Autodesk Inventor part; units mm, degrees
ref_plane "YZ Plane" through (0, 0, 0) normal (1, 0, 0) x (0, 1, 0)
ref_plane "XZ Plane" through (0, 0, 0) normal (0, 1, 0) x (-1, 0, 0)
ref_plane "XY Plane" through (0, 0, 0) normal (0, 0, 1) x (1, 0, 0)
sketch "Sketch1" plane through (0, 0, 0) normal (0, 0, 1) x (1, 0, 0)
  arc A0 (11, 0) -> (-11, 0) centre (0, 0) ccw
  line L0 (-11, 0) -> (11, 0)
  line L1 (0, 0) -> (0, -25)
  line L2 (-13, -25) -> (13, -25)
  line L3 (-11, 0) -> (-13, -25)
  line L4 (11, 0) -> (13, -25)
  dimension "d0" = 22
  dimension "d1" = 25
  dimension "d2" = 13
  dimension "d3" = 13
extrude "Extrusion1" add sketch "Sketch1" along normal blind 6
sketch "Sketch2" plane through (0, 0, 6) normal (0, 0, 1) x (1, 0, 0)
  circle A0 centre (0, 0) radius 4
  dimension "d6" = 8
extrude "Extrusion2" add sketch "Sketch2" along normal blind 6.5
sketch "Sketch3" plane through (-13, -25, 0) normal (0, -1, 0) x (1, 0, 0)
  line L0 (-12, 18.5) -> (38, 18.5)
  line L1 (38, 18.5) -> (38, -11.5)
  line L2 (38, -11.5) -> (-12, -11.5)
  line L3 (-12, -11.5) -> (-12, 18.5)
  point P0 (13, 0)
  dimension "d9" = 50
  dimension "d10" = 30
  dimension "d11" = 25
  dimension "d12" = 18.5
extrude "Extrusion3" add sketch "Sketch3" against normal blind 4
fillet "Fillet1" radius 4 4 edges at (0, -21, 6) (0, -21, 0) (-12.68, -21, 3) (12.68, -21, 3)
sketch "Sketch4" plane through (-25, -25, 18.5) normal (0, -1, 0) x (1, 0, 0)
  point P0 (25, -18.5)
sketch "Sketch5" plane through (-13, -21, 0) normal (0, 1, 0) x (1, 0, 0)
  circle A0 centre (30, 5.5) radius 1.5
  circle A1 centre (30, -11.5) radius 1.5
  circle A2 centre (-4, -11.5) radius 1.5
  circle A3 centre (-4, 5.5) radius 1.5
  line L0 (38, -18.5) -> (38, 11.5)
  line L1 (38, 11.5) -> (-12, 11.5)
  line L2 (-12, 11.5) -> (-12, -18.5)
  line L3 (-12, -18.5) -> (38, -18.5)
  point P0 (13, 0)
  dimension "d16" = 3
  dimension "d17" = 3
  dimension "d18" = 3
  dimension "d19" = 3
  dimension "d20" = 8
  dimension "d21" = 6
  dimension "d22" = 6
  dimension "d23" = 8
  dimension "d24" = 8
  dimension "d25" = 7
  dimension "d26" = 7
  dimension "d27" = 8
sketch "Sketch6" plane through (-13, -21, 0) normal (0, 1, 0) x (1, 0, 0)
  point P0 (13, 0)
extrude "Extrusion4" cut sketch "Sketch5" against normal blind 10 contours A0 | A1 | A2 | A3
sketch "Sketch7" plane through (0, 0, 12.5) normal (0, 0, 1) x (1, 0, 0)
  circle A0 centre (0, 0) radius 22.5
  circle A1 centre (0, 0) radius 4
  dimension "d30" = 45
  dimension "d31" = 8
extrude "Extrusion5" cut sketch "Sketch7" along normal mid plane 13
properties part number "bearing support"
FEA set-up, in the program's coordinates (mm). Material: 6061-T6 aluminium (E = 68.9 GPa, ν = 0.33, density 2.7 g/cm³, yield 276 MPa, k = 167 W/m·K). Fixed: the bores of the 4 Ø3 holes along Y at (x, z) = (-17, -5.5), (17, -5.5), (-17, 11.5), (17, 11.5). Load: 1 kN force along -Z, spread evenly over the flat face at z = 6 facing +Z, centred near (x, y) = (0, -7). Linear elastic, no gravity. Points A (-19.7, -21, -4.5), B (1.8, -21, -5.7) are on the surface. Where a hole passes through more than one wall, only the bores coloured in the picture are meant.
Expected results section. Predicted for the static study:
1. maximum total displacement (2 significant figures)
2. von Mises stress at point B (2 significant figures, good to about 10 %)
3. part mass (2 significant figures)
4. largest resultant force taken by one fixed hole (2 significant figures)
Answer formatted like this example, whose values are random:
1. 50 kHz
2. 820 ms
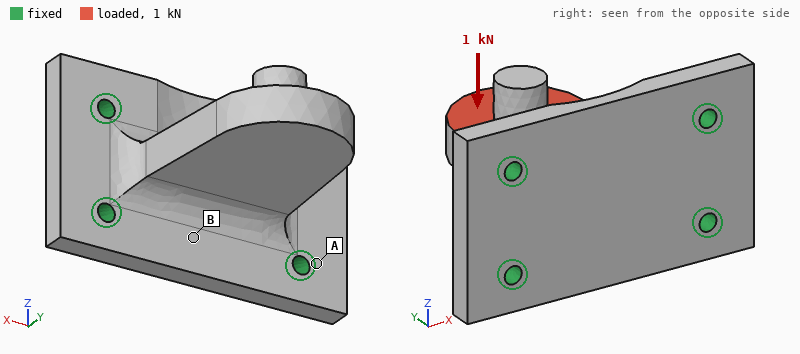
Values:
1. 0.17 mm
2. 22 MPa
3. 28 g
4. 580 N
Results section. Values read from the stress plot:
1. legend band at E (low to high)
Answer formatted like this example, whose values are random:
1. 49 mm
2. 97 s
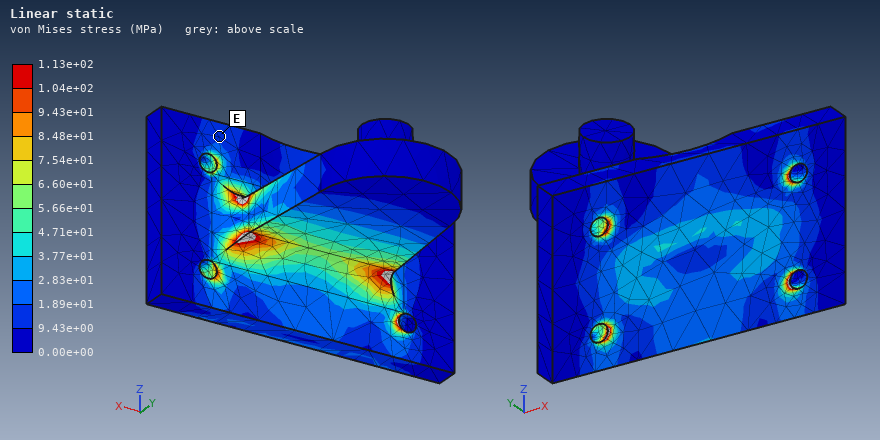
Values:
1. 9.43e+00 to 1.89e+01 MPa
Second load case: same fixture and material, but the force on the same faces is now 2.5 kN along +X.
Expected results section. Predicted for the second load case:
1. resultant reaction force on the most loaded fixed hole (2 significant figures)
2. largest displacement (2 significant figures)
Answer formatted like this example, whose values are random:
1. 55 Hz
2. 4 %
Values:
1. 1.1 kN
2. 58 µm
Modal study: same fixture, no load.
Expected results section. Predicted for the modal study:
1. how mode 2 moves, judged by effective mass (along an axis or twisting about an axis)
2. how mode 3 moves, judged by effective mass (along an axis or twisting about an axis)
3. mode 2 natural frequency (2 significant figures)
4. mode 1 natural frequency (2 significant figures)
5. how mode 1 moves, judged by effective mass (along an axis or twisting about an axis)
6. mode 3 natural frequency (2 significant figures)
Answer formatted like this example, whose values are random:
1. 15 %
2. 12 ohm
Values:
1. along X
2. along Y
3. 11 kHz
4. 4300 Hz
5. along Z
6. 15 kHz
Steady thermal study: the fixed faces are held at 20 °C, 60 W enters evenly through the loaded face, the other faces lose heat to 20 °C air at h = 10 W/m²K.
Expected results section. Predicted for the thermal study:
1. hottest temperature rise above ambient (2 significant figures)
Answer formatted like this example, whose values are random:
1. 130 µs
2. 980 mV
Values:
1. 54 K
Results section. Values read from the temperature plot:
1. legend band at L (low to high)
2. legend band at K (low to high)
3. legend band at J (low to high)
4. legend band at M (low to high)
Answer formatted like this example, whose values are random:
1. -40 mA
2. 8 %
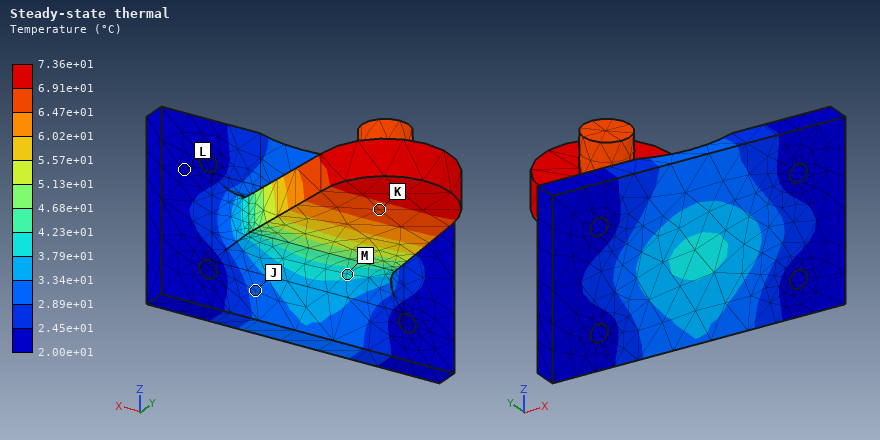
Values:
1. 2.00e+01 to 2.45e+01 °C
2. 6.47e+01 to 6.91e+01 °C
3. 2.89e+01 to 3.34e+01 °C
4. 3.79e+01 to 4.23e+01 °C
